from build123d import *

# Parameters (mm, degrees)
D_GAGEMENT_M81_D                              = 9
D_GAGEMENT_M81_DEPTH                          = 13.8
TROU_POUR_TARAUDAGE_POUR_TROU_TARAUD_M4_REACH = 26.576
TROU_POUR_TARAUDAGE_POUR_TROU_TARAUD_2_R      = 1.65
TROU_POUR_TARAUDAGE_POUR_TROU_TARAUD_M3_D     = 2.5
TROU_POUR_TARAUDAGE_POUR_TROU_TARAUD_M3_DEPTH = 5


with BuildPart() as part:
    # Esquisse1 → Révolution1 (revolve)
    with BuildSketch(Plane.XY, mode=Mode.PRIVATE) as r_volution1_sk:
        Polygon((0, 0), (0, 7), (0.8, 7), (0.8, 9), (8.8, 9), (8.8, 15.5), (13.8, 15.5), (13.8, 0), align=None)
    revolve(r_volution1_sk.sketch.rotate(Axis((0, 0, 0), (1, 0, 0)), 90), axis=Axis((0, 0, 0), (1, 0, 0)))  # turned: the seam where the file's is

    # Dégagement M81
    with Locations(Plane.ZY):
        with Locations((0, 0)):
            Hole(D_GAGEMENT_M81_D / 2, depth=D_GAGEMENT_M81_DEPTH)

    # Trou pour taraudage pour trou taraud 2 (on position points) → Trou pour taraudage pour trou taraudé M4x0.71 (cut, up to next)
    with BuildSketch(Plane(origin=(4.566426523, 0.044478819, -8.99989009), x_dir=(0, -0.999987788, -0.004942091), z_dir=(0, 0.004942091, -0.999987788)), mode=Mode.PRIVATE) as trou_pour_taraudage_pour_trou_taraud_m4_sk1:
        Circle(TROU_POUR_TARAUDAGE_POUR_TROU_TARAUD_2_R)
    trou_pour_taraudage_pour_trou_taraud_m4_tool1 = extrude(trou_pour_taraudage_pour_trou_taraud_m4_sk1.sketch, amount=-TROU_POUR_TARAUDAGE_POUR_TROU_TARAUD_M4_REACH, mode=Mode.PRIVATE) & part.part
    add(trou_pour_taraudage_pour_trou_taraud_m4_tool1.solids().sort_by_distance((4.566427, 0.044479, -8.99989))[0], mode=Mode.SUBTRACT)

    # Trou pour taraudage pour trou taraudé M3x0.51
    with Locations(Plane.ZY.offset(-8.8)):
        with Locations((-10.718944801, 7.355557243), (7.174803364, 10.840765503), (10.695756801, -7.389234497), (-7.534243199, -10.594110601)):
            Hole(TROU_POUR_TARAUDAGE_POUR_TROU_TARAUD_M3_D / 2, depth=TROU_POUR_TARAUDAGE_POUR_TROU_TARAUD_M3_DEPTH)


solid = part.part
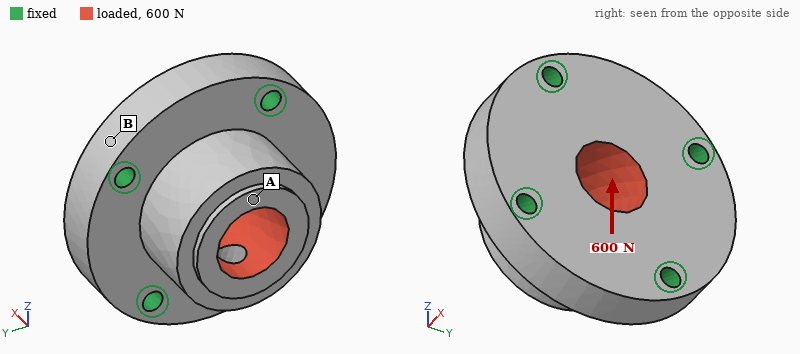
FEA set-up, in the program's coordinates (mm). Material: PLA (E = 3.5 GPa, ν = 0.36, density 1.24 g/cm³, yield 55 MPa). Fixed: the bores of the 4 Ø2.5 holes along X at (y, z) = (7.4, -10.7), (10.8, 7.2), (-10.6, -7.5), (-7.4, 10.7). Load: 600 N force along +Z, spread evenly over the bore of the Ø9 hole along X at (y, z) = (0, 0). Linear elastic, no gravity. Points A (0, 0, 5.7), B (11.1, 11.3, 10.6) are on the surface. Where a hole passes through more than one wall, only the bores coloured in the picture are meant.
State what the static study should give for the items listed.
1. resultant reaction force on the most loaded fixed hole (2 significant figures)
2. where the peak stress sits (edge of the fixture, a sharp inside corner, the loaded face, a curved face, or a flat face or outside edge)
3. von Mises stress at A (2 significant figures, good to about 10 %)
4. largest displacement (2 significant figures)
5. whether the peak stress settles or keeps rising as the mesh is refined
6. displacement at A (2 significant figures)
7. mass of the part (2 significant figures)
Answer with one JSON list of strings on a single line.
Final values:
["190 N", "edge of the fixture", "3.6 MPa", "40 µm", "keeps rising", "39 µm", "6.1 g"]
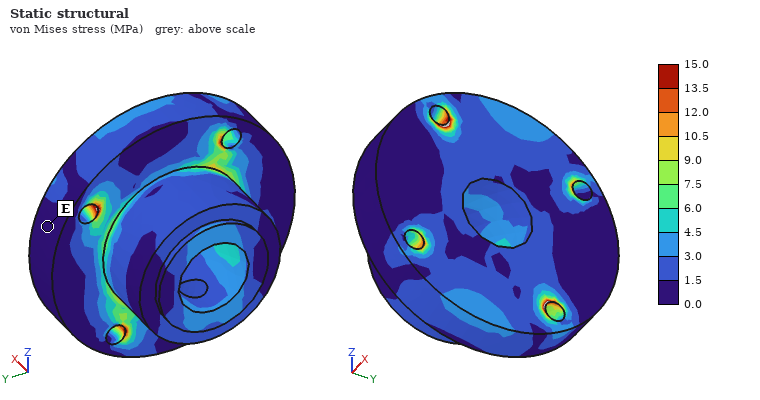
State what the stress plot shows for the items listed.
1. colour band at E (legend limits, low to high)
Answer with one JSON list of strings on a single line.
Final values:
["0.0 to 1.5 MPa"]
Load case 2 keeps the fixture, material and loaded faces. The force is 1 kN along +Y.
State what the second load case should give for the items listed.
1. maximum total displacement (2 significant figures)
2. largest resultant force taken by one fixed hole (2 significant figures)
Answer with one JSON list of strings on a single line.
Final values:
["69 µm", "320 N"]
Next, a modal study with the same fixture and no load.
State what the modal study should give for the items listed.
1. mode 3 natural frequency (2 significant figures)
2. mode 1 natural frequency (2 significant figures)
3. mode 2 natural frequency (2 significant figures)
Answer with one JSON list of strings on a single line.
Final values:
["13 kHz", "12 kHz", "12 kHz"]
